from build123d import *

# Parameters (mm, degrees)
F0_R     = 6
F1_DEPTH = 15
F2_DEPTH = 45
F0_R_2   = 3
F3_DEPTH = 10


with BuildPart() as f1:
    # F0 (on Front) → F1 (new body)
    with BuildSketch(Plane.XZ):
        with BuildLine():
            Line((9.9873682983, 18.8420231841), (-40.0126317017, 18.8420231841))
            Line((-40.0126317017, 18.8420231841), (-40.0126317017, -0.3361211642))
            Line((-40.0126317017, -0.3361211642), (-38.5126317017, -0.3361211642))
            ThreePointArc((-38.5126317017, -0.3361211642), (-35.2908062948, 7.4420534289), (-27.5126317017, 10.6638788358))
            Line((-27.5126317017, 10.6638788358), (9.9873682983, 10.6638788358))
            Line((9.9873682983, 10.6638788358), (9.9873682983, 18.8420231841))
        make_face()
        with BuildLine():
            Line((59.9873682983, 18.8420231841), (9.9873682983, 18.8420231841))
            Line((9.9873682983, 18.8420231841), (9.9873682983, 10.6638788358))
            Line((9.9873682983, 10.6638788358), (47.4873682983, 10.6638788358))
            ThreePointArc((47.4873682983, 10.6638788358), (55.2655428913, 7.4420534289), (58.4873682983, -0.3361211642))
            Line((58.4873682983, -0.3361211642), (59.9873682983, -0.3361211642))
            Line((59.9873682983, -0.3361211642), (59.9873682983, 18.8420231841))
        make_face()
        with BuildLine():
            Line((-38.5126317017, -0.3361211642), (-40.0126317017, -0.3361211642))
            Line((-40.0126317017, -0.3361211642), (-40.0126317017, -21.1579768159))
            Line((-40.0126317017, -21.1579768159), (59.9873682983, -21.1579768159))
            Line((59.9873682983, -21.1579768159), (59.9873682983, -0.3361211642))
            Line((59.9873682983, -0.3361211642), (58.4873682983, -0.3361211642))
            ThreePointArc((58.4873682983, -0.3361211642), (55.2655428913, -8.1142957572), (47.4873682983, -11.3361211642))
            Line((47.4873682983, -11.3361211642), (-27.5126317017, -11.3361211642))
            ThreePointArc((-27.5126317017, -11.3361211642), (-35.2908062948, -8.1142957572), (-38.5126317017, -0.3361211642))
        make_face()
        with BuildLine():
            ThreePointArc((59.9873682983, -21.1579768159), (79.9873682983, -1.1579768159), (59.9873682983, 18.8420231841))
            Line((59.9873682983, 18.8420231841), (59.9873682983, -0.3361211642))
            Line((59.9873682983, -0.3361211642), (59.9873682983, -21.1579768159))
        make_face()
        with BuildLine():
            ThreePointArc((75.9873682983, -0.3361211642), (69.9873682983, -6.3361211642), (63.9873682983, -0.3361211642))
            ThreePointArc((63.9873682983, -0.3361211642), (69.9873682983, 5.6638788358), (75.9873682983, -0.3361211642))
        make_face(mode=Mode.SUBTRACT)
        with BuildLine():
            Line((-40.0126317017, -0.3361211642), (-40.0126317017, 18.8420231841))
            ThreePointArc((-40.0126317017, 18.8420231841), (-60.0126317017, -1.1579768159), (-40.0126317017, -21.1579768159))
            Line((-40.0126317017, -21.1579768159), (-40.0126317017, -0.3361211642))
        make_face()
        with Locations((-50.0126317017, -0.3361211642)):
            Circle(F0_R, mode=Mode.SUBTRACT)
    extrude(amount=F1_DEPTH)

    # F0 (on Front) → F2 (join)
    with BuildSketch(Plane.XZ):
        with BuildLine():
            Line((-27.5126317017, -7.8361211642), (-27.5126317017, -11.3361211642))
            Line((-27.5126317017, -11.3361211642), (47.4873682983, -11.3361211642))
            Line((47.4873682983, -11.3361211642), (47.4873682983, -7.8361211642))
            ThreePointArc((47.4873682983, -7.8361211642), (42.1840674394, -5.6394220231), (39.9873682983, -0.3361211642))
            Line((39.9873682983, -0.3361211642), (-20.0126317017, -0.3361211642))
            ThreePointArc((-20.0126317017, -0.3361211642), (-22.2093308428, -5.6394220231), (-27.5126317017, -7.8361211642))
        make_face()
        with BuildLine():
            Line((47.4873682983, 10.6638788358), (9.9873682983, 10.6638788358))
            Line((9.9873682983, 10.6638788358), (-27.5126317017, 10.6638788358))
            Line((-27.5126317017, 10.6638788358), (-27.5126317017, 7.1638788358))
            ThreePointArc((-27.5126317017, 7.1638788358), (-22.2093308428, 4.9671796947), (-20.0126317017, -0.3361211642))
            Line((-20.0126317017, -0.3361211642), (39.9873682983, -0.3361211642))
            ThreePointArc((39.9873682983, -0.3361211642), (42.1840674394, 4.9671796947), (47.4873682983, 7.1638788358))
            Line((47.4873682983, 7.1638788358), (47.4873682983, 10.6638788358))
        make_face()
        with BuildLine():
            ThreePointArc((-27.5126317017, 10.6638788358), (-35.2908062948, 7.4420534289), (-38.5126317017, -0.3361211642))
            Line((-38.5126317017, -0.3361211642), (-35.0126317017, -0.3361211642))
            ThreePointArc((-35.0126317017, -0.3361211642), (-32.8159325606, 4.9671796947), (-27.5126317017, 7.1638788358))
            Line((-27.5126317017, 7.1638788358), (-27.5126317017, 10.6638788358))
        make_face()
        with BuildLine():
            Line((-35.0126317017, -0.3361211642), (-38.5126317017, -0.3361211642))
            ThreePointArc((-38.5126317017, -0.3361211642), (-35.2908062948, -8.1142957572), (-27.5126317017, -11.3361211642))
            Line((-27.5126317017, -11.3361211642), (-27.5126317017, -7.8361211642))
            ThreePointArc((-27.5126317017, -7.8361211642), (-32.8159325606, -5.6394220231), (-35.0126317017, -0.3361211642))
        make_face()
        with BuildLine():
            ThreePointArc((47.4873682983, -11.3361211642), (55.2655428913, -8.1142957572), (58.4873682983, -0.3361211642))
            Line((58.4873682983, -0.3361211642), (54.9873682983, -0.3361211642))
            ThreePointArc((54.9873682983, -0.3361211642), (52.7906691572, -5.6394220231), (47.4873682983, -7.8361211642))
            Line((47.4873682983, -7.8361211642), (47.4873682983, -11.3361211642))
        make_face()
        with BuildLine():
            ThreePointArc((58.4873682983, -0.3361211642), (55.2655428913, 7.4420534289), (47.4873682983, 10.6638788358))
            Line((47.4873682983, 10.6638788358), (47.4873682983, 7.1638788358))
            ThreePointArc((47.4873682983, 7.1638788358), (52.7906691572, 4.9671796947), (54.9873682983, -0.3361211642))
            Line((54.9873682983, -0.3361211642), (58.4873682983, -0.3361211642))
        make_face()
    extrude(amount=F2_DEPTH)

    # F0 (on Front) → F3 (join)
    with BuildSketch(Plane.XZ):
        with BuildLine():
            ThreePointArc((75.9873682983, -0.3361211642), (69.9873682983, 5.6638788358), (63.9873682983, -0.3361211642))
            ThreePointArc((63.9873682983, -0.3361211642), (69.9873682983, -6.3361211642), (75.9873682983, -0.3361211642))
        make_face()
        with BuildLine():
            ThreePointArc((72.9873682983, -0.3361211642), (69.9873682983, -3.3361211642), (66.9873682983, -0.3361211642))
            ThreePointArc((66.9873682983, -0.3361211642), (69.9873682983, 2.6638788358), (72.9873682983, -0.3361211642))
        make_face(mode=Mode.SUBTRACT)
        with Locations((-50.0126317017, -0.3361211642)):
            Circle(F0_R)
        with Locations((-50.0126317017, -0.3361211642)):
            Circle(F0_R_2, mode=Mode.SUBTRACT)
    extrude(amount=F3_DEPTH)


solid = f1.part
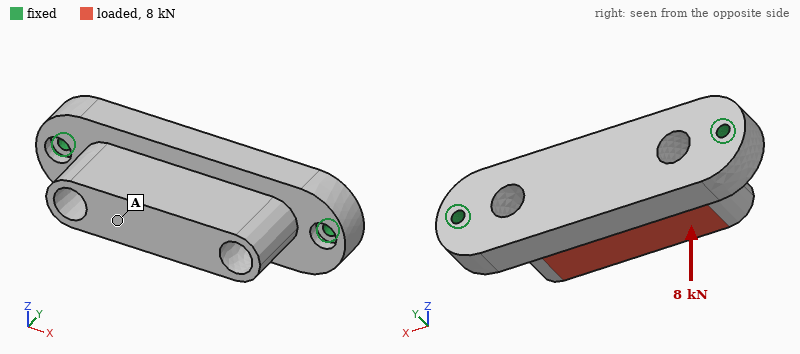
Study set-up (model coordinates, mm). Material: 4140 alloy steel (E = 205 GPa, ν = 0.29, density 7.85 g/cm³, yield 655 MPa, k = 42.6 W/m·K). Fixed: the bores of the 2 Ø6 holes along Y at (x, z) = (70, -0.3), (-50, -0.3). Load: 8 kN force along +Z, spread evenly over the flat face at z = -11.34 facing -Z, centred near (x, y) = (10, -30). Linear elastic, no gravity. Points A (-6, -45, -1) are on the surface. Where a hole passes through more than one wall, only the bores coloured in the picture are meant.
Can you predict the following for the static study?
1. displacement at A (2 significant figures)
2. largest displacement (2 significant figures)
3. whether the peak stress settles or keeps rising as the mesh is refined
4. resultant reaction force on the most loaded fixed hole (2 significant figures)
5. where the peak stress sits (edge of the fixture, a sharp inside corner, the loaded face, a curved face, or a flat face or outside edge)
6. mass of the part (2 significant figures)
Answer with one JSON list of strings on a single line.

["87 µm", "90 µm", "keeps rising", "4.0 kN", "edge of the fixture", "960 g"]
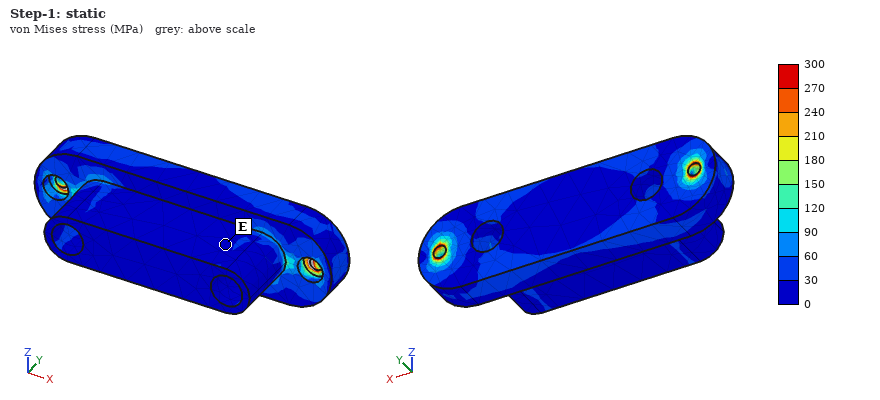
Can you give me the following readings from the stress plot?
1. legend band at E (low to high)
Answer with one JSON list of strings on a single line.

["0 to 30 MPa"]
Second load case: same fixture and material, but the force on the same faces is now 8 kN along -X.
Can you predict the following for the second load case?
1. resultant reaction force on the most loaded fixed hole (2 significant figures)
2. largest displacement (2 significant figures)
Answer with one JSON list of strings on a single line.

["4.4 kN", "7.0 µm"]
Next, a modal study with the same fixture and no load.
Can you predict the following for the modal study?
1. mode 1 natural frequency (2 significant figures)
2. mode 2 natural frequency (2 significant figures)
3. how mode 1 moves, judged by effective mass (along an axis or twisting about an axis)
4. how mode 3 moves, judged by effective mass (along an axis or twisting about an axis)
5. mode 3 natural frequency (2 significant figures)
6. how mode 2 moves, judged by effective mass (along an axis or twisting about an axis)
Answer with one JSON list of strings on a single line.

["2600 Hz", "4700 Hz", "along Z", "along Z", "5800 Hz", "along Y"]
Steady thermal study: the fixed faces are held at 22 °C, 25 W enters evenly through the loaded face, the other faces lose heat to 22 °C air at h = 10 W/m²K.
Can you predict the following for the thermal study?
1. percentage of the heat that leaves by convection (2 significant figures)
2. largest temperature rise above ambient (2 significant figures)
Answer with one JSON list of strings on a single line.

["15 %", "28 K"]
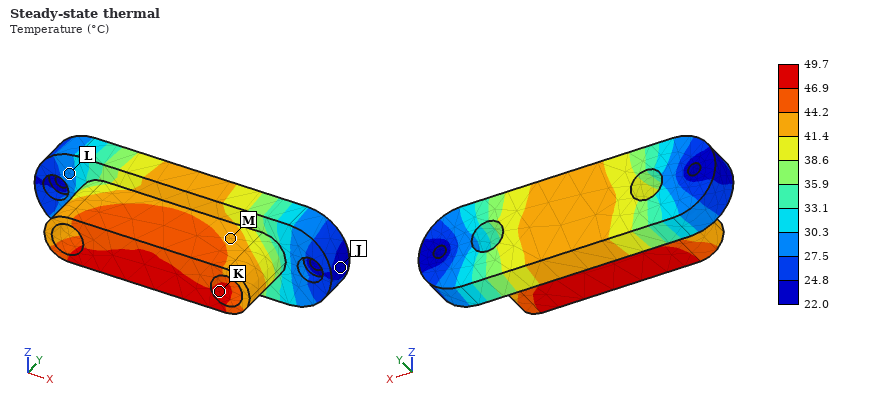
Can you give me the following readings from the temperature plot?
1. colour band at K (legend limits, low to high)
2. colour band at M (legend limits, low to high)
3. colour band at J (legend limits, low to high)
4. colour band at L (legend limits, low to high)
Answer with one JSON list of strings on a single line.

["46.9 to 49.7 °C", "41.4 to 44.2 °C", "22.0 to 24.8 °C", "27.5 to 30.3 °C"]
